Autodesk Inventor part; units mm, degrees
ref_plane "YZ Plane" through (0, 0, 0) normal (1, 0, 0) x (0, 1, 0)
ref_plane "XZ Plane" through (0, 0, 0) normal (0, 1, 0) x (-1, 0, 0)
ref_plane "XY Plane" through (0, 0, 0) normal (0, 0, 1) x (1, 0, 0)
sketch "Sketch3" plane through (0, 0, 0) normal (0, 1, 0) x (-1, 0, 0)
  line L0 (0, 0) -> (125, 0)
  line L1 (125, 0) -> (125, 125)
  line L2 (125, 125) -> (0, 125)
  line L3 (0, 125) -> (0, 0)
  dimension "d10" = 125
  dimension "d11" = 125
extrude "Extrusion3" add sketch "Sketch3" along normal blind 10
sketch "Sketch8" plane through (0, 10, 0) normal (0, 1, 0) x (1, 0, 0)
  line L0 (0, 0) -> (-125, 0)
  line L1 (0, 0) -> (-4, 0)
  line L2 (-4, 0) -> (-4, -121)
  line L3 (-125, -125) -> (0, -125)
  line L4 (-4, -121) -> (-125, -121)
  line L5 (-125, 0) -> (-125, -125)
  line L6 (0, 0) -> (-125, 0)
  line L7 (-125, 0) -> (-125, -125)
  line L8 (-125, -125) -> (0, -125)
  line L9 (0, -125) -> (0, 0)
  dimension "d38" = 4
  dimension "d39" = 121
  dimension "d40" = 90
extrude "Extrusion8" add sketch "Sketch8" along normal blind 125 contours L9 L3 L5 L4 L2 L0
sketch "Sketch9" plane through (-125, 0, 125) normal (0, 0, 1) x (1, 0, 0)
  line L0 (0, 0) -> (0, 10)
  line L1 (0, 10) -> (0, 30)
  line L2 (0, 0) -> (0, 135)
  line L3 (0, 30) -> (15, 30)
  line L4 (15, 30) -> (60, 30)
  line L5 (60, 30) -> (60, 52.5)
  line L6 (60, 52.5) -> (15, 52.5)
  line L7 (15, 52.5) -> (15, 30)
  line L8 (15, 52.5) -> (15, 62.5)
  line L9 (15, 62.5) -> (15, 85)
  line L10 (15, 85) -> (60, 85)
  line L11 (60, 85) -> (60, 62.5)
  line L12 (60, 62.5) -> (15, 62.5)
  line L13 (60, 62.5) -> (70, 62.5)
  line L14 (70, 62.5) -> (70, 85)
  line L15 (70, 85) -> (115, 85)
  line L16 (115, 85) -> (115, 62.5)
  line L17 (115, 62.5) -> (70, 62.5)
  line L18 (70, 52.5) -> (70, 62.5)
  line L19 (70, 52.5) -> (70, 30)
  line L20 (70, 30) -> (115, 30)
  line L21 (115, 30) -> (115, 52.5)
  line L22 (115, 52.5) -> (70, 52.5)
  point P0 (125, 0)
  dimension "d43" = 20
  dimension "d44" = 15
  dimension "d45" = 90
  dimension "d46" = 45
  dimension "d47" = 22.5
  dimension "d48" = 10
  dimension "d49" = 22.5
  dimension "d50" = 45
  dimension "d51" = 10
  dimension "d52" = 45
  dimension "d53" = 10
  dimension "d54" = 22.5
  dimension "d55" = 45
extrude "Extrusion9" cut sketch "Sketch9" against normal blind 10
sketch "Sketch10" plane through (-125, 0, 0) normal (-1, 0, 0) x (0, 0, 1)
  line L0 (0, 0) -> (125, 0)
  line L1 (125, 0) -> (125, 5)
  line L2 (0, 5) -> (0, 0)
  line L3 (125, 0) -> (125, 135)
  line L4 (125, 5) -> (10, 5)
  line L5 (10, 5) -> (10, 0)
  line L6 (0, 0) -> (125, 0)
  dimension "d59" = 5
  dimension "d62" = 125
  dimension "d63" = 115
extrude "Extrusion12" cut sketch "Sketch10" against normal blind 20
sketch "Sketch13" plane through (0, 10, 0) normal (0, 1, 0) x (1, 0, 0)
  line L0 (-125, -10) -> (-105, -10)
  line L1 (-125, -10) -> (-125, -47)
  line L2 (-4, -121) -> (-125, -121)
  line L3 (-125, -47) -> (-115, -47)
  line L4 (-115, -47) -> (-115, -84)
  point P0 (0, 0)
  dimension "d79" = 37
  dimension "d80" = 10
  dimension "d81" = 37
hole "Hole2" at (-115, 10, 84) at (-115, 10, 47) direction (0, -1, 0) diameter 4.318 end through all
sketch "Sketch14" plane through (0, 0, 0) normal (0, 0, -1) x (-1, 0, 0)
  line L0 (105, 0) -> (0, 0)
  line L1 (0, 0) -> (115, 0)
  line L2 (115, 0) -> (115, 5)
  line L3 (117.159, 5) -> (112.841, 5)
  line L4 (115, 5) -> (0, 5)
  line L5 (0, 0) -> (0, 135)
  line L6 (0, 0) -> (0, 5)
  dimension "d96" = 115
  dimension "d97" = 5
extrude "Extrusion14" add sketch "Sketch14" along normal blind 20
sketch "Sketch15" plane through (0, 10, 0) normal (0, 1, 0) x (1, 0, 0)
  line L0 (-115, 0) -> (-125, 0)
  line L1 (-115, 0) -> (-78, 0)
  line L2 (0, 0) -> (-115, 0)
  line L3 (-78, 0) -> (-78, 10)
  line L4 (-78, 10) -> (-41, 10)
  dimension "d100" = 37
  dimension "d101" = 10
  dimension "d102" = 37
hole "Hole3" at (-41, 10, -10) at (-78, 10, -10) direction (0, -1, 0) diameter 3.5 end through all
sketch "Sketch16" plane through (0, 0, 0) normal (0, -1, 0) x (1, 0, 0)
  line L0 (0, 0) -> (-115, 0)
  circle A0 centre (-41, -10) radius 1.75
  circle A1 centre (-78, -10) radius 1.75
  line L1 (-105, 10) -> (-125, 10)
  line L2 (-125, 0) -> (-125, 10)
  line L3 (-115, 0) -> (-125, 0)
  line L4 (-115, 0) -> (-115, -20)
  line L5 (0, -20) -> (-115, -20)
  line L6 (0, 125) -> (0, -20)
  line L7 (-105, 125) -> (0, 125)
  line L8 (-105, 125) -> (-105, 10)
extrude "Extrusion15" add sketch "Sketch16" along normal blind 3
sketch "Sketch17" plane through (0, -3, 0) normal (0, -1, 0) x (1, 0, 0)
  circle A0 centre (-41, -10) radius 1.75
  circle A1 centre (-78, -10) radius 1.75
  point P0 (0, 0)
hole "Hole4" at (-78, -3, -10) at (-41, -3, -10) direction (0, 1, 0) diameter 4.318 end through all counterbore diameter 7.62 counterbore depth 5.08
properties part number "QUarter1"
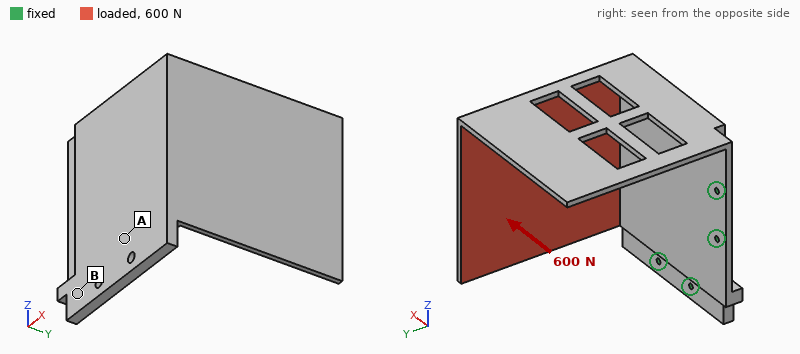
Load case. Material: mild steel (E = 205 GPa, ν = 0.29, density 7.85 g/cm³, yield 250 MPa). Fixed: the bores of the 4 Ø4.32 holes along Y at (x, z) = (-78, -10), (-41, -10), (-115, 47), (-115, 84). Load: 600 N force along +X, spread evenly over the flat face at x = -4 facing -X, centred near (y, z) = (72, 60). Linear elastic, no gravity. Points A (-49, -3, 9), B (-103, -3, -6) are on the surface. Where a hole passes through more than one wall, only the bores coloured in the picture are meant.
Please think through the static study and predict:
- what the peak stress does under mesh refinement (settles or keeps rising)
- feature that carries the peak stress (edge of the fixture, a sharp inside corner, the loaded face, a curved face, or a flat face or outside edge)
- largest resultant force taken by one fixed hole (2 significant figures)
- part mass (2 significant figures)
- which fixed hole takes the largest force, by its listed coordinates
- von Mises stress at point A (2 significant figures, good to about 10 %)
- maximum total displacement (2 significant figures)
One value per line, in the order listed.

keeps rising
edge of the fixture
880 N
2.4 kg
(-41, -10)
17 MPa
0.60 mm
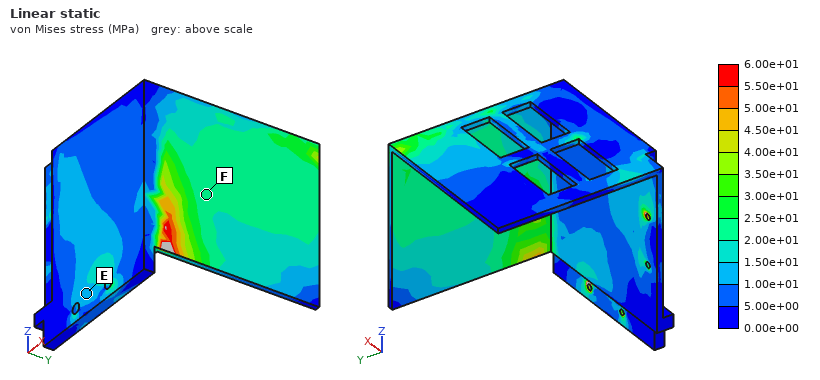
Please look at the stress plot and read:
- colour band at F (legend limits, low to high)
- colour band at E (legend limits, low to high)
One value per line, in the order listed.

2.00e+01 to 2.50e+01 MPa
1.00e+01 to 1.50e+01 MPa
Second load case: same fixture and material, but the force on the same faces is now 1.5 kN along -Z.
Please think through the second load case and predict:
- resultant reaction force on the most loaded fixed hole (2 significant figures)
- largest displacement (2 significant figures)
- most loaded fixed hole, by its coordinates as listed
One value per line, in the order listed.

2.5 kN
0.42 mm
(-41, -10)
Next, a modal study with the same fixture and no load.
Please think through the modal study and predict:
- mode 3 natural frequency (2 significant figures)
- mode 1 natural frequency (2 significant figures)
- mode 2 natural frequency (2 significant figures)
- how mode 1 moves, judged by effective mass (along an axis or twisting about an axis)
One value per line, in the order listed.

460 Hz
260 Hz
290 Hz
along Y
